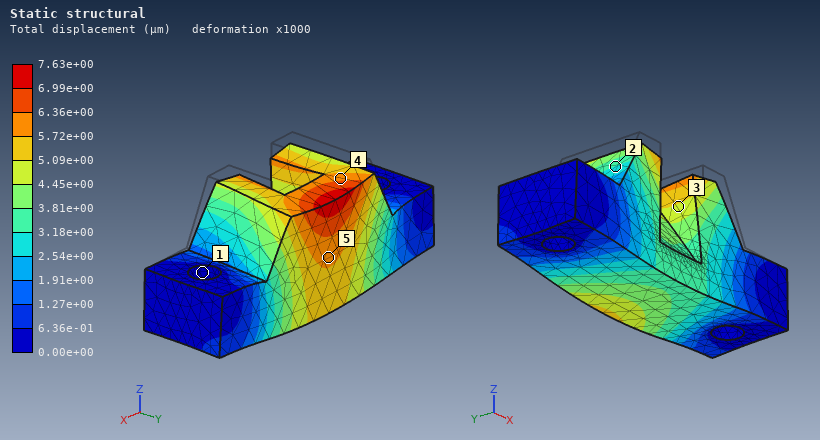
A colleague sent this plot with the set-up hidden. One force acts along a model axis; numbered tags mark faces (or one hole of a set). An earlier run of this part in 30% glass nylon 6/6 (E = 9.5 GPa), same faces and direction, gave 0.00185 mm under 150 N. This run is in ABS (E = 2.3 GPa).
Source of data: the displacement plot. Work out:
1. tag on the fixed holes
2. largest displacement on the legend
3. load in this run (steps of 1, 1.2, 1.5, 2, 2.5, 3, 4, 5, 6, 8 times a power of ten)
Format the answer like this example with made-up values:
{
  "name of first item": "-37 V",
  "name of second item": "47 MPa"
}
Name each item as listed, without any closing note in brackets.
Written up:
{
  "tag on the fixed holes": "1",
  "largest displacement on the legend": "7.63e+00 µm",
  "load in this run": "150 N"
}
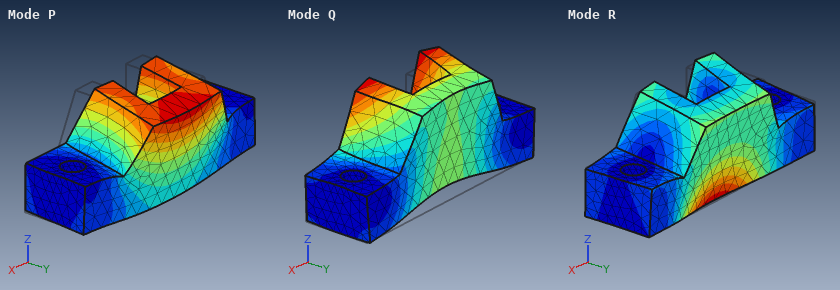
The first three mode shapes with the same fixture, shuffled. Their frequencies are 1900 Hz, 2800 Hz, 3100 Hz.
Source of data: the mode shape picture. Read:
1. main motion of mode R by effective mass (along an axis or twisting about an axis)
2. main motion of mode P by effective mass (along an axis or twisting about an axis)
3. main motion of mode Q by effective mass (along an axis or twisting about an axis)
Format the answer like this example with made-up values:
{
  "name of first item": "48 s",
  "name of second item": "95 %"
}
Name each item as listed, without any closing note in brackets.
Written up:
{
  "main motion of mode R by effective mass": "along Y",
  "main motion of mode P by effective mass": "along Y",
  "main motion of mode Q by effective mass": "along Z"
}
